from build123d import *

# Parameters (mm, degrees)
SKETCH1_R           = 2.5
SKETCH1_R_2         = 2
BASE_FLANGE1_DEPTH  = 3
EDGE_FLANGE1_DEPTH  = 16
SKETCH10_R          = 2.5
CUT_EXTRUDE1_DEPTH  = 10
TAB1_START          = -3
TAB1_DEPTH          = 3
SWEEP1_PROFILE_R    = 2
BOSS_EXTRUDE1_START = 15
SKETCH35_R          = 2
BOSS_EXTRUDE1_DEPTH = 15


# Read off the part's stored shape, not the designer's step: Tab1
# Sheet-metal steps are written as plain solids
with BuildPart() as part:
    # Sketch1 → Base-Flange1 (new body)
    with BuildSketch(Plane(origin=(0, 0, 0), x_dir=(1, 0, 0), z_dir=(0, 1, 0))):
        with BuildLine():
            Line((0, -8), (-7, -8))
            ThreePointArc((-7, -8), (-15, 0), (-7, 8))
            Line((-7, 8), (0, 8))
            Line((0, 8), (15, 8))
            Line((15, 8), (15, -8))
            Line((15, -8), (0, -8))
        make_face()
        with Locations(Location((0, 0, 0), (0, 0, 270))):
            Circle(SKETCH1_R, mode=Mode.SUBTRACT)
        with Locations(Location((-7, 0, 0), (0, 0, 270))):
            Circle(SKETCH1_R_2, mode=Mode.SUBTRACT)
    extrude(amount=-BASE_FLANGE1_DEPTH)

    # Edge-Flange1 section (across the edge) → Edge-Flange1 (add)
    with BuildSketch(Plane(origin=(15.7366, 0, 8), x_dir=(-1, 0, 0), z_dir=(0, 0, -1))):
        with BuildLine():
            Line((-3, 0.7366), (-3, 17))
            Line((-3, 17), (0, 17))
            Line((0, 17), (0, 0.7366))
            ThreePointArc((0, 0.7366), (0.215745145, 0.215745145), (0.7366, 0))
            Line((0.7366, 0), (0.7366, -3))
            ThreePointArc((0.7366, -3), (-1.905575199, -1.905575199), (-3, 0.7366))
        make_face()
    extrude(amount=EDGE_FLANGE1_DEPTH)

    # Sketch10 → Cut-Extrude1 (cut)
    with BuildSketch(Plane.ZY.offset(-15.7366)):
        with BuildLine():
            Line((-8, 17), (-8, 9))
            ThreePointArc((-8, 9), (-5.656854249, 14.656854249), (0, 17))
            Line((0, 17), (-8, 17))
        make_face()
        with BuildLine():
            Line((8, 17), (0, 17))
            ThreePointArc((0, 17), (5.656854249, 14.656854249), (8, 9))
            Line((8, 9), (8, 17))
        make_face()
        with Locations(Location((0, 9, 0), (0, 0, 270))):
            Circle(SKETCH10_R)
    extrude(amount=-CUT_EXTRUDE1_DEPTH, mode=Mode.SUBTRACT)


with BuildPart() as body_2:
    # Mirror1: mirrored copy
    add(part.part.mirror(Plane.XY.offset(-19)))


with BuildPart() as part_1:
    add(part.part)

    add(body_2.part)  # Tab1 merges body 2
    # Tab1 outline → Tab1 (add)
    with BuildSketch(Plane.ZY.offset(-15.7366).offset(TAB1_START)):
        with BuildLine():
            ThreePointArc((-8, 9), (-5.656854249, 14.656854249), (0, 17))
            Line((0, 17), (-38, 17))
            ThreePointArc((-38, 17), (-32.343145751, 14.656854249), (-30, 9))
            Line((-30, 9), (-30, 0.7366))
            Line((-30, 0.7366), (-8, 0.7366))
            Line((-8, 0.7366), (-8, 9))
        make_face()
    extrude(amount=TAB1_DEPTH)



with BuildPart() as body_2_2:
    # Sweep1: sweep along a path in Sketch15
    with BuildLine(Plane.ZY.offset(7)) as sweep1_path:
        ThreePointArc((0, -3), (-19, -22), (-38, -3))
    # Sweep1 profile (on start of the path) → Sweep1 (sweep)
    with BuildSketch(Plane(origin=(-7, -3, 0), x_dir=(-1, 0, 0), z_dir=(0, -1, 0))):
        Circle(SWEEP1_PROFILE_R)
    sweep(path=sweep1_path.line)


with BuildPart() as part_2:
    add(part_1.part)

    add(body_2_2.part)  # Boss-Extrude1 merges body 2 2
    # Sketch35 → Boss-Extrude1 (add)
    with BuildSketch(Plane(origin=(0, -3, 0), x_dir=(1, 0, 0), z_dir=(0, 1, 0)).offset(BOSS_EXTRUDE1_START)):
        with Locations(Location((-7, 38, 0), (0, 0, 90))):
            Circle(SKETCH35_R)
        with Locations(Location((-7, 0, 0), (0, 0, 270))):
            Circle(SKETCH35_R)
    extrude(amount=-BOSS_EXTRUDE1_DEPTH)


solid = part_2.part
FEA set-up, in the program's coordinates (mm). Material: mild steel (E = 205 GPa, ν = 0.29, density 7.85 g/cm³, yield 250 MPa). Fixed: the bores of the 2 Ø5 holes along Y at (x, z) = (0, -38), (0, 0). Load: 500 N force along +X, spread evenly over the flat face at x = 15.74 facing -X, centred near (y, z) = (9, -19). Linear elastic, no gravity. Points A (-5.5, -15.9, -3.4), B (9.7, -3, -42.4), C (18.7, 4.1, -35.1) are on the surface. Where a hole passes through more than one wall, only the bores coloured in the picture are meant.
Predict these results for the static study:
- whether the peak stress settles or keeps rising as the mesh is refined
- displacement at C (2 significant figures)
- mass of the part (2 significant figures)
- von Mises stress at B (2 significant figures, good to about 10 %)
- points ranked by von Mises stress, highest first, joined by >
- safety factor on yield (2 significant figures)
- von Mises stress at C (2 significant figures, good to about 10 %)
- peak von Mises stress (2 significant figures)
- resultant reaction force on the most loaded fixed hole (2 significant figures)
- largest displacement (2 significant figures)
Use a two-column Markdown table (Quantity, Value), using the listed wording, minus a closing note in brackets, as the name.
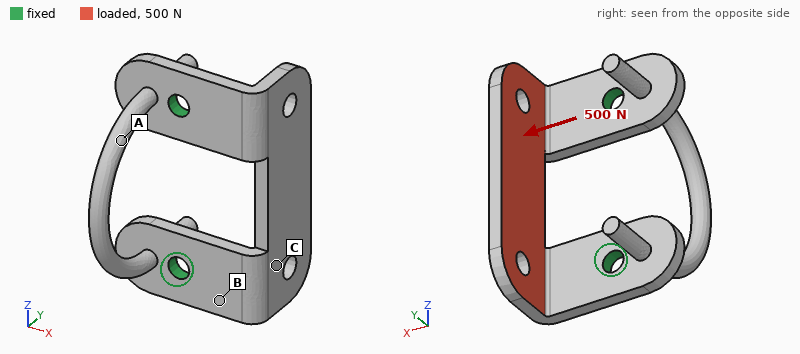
| Quantity | Value |
|---|---|
| whether the peak stress settles or keeps rising as the mesh is refined | settles |
| displacement at C | 0.062 mm |
| mass of the part | 50 g |
| von Mises stress at B | 95 MPa |
| points ranked by von Mises stress, highest first, joined by > | B > C > A |
| safety factor on yield | 0.76 |
| von Mises stress at C | 52 MPa |
| peak von Mises stress | 330 MPa |
| resultant reaction force on the most loaded fixed hole | 250 N |
| largest displacement | 0.14 mm |
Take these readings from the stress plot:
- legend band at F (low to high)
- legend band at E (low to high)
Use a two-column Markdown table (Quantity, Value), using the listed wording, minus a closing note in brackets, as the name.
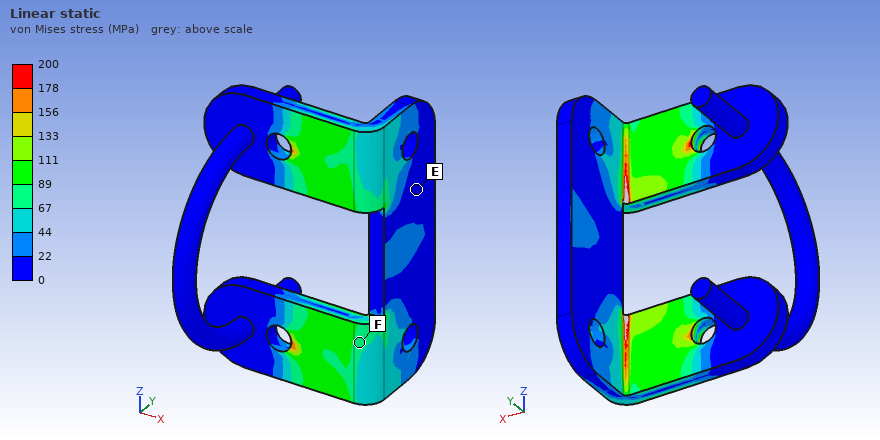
| Quantity | Value |
|---|---|
| legend band at F | 67 to 89 MPa |
| legend band at E | 0 to 22 MPa |
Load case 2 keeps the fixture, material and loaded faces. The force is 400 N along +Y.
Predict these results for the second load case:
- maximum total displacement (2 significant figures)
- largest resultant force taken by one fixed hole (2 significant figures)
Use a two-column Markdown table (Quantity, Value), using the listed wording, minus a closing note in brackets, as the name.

| Quantity | Value |
|---|---|
| maximum total displacement | 59 µm |
| largest resultant force taken by one fixed hole | 200 N |
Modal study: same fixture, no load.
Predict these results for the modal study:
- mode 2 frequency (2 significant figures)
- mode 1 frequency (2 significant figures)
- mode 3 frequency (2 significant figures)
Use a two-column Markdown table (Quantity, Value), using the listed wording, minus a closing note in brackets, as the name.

| Quantity | Value |
|---|---|
| mode 2 frequency | 3300 Hz |
| mode 1 frequency | 2300 Hz |
| mode 3 frequency | 4200 Hz |
